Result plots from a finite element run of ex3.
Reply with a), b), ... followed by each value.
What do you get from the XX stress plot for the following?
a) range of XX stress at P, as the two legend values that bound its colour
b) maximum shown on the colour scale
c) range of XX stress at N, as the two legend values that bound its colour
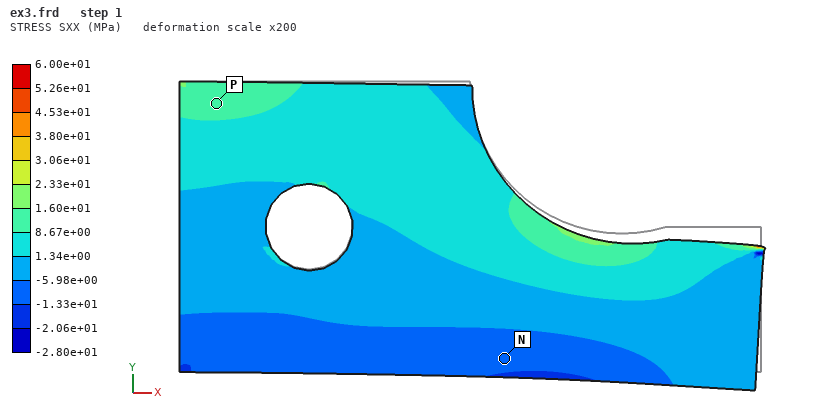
a) 8.67e+00 to 1.60e+01 MPa
b) 6.00e+01 MPa
c) -1.33e+01 to -5.98e+00 MPa
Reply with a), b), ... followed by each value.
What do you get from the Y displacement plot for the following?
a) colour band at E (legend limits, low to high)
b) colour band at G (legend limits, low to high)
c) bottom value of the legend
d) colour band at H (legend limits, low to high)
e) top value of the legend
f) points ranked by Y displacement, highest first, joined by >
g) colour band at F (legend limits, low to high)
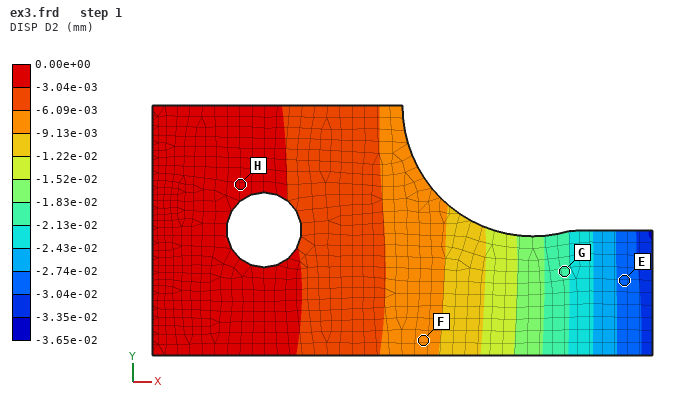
a) -3.04e-02 to -2.74e-02 mm
b) -2.13e-02 to -1.83e-02 mm
c) -3.65e-02 mm
d) -3.04e-03 to 0.00e+00 mm
e) 0.00e+00 mm
f) H > F > G > E
g) -9.13e-03 to -6.09e-03 mm
